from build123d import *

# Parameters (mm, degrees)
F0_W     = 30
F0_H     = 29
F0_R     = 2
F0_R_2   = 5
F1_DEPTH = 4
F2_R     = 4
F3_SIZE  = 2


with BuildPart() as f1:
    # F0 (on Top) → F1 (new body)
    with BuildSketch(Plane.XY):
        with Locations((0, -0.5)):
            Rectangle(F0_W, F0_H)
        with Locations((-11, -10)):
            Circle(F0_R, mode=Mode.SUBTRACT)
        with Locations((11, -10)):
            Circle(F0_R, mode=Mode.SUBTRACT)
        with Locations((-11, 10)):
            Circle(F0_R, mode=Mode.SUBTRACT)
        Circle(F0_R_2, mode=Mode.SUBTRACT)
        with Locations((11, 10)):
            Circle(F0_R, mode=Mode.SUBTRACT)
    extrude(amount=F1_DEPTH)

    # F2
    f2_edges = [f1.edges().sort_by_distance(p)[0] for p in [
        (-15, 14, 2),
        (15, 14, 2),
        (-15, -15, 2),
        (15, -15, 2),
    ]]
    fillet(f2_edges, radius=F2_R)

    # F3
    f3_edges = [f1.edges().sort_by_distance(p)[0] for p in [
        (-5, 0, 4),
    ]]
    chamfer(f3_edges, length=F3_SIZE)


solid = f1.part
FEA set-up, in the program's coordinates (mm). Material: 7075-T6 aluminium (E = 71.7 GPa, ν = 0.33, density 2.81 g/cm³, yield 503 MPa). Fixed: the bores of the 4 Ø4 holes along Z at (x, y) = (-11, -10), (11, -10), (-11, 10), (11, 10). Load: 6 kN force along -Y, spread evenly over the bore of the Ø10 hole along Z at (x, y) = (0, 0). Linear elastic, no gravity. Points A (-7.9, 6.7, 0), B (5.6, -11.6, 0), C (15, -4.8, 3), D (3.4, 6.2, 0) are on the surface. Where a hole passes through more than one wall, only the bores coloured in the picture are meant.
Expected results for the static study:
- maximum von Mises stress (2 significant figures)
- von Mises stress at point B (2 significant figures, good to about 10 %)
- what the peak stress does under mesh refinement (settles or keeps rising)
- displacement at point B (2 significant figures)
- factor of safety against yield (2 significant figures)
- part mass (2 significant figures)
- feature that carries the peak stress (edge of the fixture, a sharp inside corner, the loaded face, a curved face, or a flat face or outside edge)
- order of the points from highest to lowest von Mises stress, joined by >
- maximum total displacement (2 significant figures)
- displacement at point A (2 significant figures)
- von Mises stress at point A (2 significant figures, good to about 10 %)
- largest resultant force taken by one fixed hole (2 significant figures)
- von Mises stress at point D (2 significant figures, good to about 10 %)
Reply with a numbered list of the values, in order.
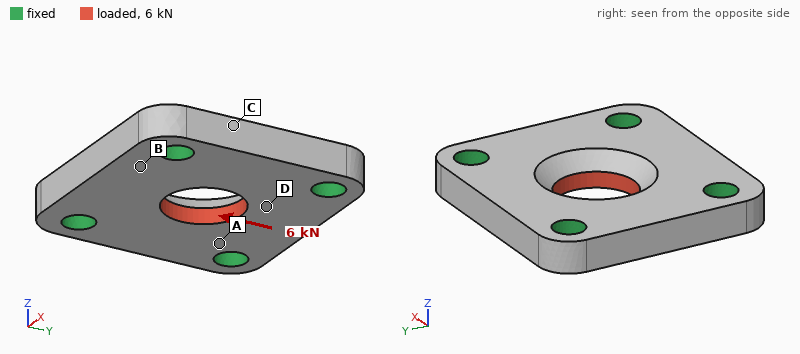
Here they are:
1. 190 MPa
2. 44 MPa
3. settles
4. 5.6 µm
5. 2.7
6. 8.0 g
7. the loaded face
8. D > A > B > C
9. 16 µm
10. 3.2 µm
11. 69 MPa
12. 1.6 kN
13. 91 MPa
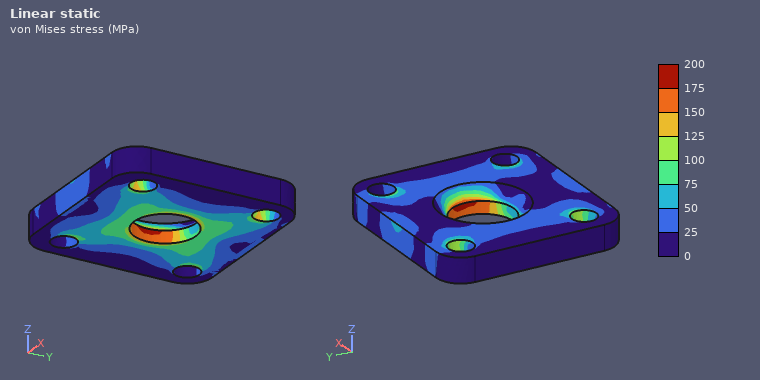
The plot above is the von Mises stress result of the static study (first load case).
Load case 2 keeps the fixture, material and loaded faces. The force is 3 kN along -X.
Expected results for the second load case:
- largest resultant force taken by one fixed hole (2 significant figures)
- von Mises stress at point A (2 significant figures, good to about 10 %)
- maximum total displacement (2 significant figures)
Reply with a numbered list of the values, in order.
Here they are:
1. 810 N
2. 36 MPa
3. 7.2 µm
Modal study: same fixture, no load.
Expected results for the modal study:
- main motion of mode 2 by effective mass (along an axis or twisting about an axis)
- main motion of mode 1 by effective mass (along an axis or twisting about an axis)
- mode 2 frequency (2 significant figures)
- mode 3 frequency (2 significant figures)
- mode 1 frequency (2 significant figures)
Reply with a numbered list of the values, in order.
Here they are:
1. twisting about X
2. along Z
3. 44 kHz
4. 49 kHz
5. 39 kHz
